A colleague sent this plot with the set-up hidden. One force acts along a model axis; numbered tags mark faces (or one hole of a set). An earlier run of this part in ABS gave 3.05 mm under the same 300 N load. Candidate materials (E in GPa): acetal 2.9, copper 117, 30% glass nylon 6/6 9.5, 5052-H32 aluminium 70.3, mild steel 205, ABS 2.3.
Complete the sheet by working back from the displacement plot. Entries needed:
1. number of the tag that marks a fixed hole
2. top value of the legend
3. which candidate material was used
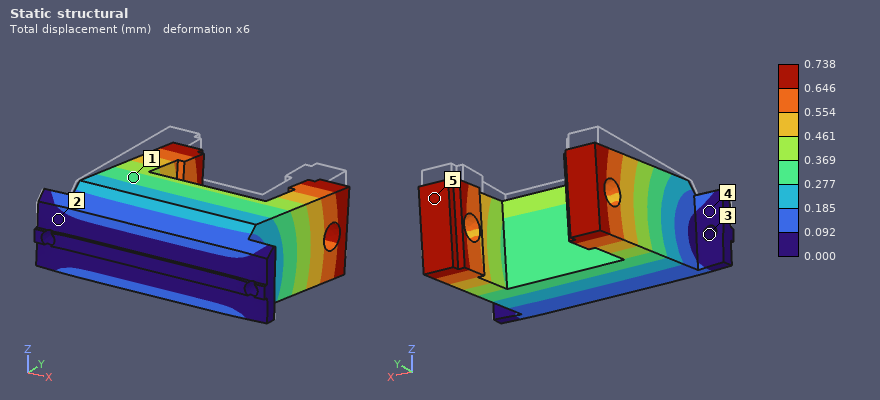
3
0.738 mm
30% glass nylon 6/6
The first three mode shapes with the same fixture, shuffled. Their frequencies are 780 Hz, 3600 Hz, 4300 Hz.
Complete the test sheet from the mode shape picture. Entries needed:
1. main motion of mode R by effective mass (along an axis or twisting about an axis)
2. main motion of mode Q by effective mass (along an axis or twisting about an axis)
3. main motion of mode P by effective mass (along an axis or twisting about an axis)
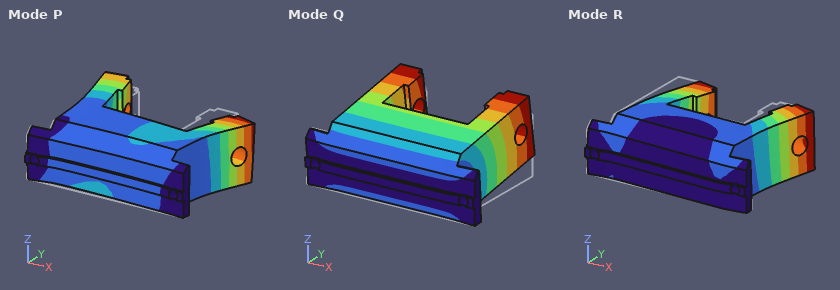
along X
along Z
along Y
